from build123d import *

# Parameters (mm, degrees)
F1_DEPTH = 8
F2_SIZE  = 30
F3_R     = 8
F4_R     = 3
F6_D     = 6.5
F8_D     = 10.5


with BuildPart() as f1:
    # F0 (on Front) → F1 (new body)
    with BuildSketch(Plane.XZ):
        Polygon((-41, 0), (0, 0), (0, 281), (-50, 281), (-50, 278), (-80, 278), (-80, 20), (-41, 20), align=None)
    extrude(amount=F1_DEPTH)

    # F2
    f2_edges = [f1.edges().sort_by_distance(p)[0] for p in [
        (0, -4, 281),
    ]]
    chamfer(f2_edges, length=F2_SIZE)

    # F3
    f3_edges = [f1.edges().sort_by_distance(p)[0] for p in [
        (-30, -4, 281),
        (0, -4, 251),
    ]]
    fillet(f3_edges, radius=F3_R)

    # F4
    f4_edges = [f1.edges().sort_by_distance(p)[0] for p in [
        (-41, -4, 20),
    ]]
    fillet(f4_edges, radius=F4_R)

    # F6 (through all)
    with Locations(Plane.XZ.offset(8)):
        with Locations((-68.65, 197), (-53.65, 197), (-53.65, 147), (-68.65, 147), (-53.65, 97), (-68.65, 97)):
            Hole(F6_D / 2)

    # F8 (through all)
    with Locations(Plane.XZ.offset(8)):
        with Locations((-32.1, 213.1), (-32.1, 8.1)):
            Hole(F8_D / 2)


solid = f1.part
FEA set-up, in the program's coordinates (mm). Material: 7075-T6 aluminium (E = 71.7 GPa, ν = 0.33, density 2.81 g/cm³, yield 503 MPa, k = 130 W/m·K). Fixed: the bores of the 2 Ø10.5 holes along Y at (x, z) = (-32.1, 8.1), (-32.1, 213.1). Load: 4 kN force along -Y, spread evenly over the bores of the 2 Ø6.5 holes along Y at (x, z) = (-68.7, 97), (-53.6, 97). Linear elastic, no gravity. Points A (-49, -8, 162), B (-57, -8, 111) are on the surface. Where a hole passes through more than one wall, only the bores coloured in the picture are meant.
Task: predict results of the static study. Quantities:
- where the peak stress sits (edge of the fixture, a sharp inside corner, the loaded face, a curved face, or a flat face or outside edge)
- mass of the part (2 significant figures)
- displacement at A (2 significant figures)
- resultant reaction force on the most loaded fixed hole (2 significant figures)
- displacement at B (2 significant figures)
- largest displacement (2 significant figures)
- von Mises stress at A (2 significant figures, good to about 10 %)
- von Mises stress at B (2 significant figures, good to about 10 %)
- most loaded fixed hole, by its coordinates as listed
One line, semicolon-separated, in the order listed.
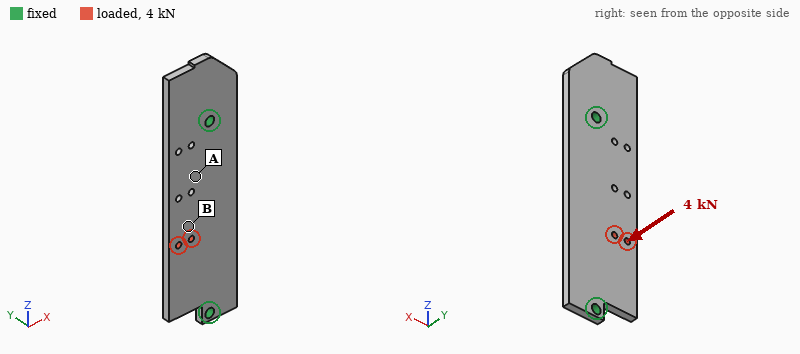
a curved face; 470 g; 0.56 mm; 2.2 kN; 1.2 mm; 1.7 mm; 54 MPa; 110 MPa; (-32.1, 8.1)
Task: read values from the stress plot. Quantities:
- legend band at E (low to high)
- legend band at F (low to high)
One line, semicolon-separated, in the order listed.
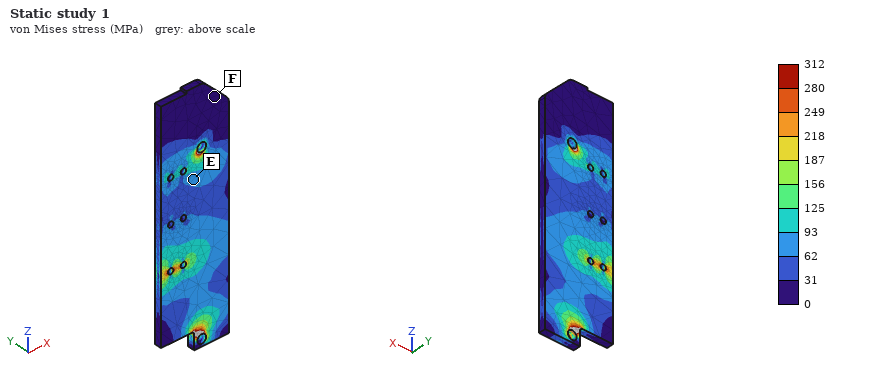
62 to 93 MPa; 0 to 31 MPa
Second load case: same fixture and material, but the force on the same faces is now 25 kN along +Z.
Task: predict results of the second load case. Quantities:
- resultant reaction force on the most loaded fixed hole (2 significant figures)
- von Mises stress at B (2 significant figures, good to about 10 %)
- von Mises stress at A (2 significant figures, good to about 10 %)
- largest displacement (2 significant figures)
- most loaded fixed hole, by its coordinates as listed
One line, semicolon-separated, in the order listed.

14 kN; 52 MPa; 28 MPa; 68 µm; (-32.1, 213.1)
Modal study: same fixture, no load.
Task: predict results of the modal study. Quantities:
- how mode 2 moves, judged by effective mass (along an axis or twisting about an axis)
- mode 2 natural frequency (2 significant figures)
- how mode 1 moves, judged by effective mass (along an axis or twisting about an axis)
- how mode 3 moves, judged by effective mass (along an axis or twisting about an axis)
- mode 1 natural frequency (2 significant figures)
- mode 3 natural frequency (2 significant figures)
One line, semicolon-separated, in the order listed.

twisting about Z; 1300 Hz; along Y; along Y; 840 Hz; 1500 Hz
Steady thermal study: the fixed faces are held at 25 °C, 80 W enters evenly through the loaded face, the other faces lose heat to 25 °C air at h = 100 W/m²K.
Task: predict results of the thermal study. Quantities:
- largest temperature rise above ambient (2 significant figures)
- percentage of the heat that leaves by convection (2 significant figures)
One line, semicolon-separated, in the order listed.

48 K; 68 %
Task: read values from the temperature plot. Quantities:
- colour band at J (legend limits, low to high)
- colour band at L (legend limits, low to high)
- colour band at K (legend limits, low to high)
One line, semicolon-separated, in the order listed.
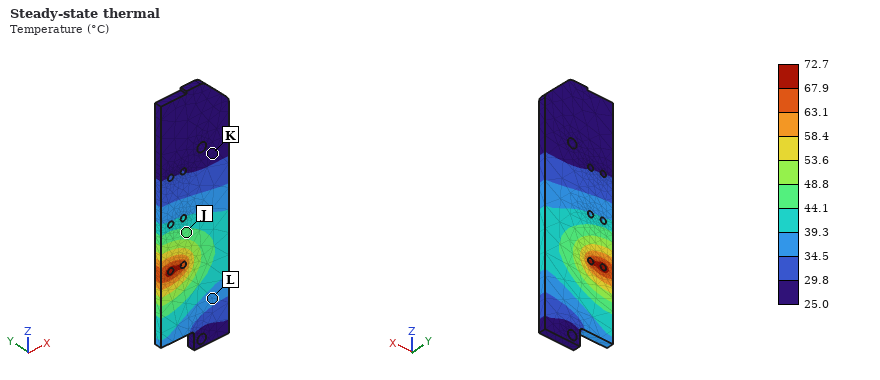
44.1 to 48.8 °C; 34.5 to 39.3 °C; 25.0 to 29.8 °C
